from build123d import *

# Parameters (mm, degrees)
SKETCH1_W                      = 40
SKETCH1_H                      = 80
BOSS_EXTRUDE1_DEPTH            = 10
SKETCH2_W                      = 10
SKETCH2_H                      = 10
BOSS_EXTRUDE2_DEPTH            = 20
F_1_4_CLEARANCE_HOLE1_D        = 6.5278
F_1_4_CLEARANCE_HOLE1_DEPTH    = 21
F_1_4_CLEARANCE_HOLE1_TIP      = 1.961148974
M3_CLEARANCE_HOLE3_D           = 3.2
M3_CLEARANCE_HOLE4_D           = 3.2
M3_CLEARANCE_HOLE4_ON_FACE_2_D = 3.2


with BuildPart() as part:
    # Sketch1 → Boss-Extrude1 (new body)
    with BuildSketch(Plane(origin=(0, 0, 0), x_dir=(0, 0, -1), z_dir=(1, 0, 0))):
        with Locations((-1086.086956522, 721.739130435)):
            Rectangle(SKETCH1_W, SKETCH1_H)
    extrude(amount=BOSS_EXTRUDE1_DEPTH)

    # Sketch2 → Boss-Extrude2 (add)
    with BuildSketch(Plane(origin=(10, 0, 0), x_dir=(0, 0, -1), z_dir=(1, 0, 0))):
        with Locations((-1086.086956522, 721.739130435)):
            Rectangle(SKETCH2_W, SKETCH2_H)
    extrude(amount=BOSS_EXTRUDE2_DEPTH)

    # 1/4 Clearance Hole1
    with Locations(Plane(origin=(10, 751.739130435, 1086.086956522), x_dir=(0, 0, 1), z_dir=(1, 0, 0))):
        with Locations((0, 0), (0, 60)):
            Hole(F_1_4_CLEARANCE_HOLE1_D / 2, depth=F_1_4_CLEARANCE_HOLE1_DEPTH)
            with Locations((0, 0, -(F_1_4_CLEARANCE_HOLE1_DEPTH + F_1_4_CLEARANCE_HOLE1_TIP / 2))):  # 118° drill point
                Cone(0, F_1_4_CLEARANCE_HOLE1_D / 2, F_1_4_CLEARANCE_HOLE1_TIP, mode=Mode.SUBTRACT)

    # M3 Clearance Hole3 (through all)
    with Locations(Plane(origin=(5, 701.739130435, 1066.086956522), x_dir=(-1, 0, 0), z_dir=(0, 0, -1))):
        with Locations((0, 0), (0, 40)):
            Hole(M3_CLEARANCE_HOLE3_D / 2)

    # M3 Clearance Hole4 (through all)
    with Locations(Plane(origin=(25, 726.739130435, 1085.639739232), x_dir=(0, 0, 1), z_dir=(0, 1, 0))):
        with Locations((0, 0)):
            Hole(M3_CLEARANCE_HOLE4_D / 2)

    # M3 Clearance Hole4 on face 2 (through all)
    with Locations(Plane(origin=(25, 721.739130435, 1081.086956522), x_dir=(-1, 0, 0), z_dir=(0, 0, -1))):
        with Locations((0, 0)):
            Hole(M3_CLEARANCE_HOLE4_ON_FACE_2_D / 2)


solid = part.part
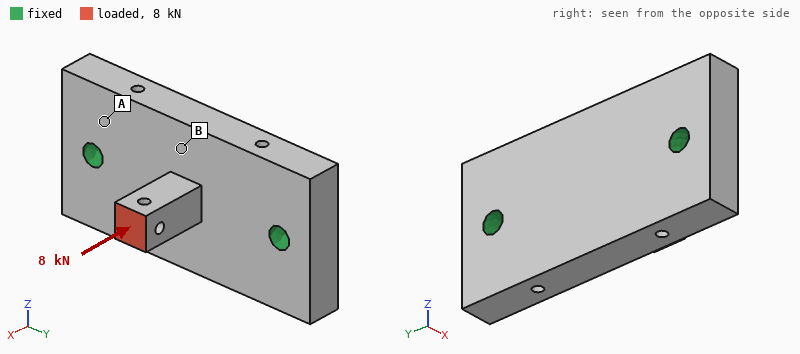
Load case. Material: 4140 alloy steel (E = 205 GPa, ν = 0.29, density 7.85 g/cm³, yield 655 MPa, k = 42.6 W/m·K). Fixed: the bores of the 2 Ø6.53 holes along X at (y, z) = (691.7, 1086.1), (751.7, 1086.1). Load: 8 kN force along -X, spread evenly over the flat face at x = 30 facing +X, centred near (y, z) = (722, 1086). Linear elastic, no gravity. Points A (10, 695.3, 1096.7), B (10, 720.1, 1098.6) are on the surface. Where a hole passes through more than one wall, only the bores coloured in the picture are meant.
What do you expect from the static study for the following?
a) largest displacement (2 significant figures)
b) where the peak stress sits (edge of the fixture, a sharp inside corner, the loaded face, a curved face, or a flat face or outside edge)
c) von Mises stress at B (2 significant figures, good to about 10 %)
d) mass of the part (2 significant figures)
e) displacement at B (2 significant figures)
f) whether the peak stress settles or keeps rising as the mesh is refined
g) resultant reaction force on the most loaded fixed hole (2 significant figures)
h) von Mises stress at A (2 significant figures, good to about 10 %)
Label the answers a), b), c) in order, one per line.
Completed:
a) 32 µm
b) a sharp inside corner
c) 60 MPa
d) 260 g
e) 19 µm
f) keeps rising
g) 4.0 kN
h) 31 MPa
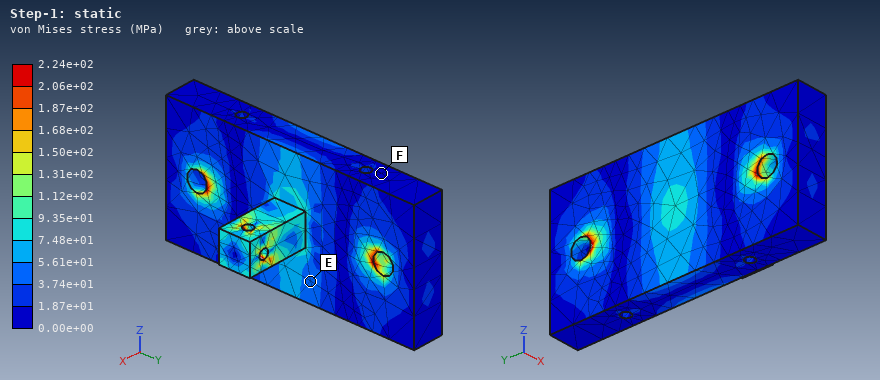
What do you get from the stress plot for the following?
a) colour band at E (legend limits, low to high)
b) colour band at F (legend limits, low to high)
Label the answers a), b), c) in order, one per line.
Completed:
a) 3.74e+01 to 5.61e+01 MPa
b) 0.00e+00 to 1.87e+01 MPa
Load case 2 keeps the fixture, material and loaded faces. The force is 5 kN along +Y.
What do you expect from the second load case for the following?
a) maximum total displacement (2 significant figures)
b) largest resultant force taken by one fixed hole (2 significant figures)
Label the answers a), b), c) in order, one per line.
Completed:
a) 0.15 mm
b) 3.7 kN
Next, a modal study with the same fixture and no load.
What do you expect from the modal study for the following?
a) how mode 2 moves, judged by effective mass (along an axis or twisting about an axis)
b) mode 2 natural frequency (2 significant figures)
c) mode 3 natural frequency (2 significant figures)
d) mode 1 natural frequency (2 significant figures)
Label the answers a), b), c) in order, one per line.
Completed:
a) along X
b) 9700 Hz
c) 14 kHz
d) 9100 Hz
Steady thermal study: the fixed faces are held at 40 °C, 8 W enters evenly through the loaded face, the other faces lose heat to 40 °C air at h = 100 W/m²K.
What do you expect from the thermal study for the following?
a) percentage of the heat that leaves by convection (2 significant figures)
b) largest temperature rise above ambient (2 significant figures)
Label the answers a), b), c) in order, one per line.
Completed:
a) 51 %
b) 46 K
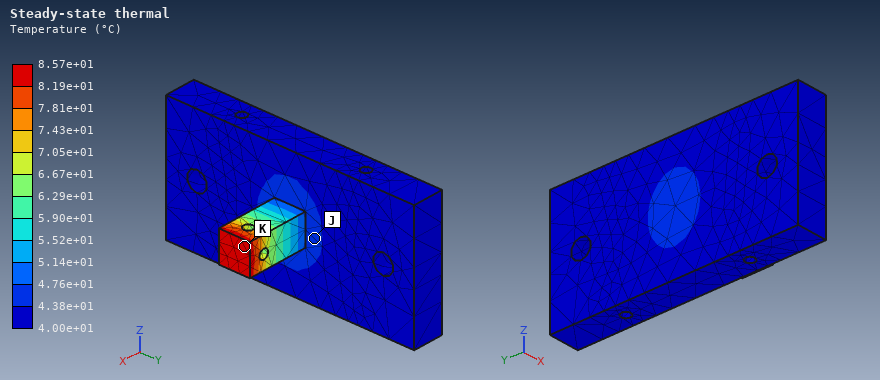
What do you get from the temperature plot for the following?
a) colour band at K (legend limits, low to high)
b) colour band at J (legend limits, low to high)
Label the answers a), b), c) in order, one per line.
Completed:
a) 8.19e+01 to 8.57e+01 °C
b) 4.38e+01 to 4.76e+01 °C
